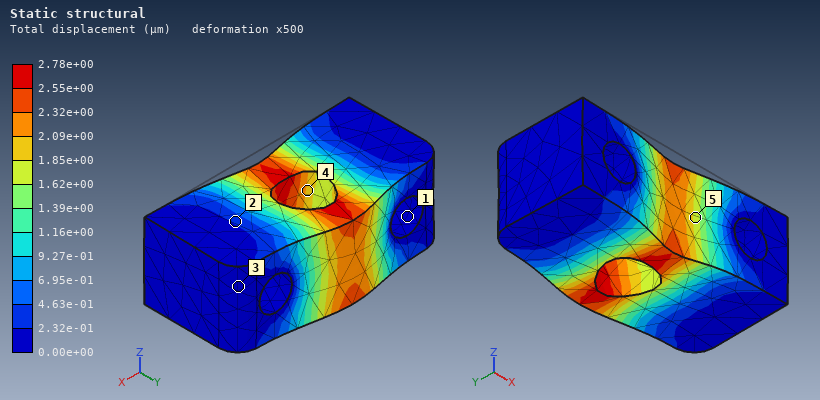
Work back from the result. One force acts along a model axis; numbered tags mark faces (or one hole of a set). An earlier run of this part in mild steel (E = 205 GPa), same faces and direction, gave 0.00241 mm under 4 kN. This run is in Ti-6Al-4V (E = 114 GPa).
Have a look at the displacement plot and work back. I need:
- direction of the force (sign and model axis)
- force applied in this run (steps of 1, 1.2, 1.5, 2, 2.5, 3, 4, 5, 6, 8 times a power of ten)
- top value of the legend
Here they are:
+Y
2.5 kN
2.78e+00 µm
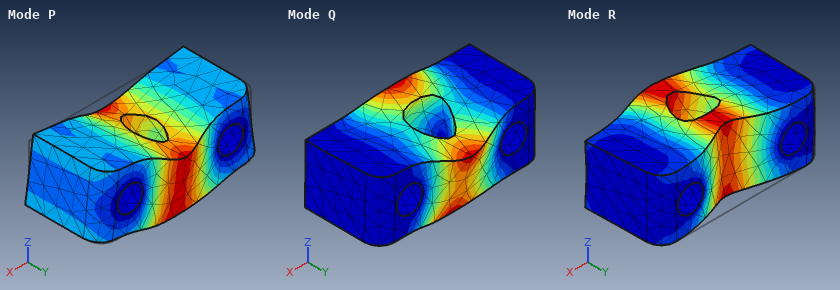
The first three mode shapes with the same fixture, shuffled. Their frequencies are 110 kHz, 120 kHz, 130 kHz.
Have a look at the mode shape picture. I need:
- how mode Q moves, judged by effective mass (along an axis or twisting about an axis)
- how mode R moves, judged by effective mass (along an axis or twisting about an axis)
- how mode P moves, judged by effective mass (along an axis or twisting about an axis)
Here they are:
twisting about X
along Y
along Z
